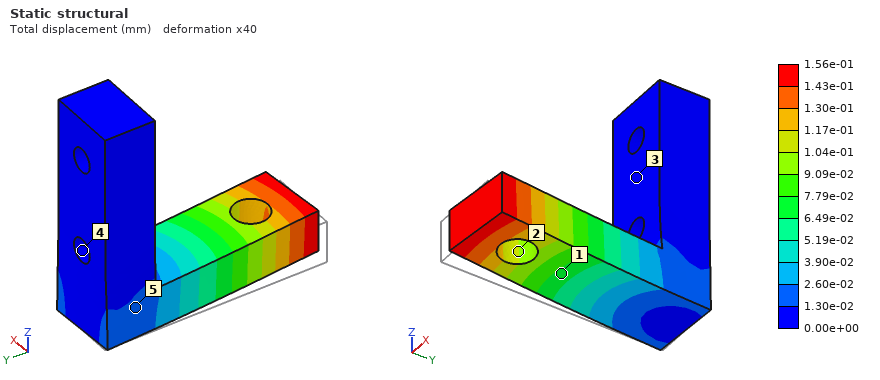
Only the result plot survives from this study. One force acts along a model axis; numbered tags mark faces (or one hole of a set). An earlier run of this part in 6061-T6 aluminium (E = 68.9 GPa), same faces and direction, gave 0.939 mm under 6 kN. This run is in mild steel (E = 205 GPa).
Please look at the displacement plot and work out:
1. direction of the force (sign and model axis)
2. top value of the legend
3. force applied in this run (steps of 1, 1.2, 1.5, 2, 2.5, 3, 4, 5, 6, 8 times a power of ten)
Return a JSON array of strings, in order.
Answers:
["+X", "1.56e-01 mm", "3 kN"]
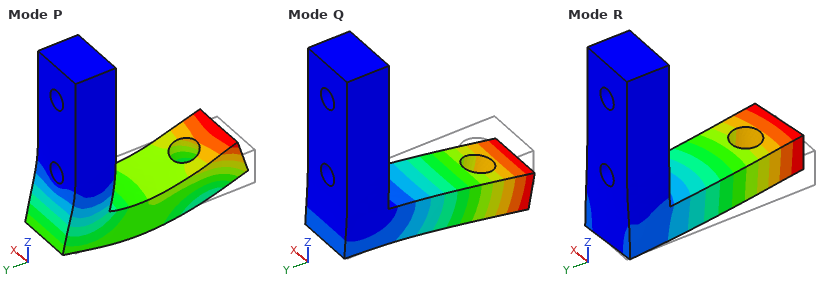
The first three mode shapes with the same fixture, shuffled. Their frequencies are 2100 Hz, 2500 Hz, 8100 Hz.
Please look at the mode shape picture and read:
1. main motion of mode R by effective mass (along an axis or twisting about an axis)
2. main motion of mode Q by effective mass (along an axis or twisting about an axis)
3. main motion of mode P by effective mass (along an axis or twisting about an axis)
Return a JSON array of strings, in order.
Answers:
["along X", "along Z", "along Y"]
